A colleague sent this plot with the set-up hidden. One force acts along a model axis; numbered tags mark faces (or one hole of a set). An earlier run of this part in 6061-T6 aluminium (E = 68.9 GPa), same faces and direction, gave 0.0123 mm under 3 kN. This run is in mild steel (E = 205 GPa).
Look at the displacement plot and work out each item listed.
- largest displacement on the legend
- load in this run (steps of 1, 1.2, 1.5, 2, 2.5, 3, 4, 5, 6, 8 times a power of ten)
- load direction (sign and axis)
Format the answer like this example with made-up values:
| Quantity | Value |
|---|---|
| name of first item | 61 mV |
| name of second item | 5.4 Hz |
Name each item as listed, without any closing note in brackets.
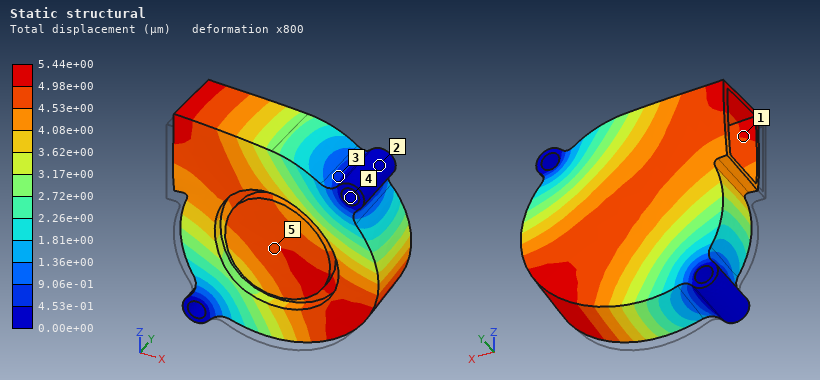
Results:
| Quantity | Value |
|---|---|
| largest displacement on the legend | 5.44e+00 µm |
| load in this run | 4 kN |
| load direction | +Y |
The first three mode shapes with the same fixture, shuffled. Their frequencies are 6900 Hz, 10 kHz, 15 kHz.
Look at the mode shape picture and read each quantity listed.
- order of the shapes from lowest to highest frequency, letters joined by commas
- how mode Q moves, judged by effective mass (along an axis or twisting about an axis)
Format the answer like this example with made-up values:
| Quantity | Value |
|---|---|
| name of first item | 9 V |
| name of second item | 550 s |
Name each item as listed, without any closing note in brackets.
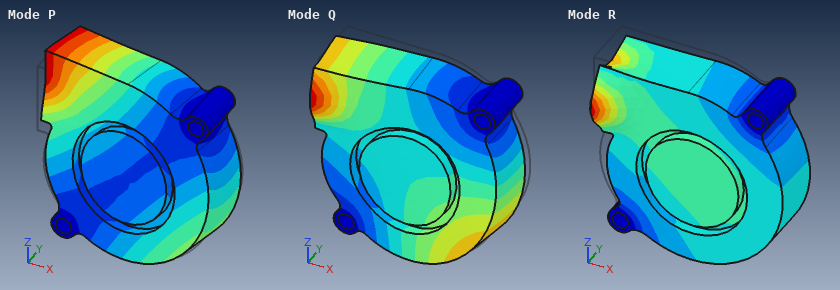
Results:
| Quantity | Value |
|---|---|
| order of the shapes from lowest to highest frequency, letters joined by commas | P, Q, R |
| how mode Q moves, judged by effective mass | along Y |
